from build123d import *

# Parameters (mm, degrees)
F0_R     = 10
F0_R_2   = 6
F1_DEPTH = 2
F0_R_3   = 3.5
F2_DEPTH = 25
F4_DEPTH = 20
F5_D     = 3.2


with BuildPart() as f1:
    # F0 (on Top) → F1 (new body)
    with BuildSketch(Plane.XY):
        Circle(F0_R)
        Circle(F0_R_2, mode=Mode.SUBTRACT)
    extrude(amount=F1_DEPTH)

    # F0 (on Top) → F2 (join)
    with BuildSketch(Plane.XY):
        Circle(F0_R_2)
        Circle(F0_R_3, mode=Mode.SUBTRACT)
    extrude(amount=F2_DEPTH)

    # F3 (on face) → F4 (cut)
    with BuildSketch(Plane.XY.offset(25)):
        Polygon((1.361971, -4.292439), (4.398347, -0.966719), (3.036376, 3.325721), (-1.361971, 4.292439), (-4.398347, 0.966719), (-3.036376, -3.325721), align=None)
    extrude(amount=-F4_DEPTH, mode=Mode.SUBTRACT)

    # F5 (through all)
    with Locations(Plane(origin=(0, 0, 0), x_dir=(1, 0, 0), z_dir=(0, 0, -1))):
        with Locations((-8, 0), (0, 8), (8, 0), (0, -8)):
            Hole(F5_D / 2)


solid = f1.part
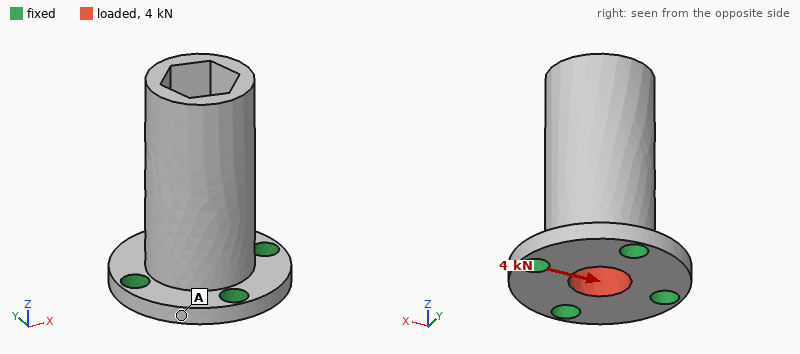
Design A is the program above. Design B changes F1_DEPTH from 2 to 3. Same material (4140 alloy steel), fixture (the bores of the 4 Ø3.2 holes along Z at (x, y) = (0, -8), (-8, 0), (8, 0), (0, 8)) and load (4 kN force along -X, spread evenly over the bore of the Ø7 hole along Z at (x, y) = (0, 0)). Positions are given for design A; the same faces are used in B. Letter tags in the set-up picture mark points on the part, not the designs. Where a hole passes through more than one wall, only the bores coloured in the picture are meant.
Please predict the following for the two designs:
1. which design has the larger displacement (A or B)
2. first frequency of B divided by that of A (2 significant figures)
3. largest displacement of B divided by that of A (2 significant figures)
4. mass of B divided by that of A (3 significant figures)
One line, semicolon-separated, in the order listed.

A; 1.1; 0.44; 1.09
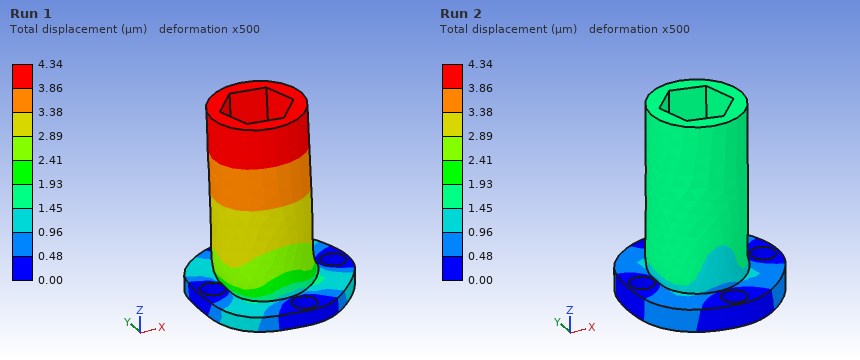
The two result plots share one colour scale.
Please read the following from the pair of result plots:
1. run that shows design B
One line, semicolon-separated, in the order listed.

Run 2
